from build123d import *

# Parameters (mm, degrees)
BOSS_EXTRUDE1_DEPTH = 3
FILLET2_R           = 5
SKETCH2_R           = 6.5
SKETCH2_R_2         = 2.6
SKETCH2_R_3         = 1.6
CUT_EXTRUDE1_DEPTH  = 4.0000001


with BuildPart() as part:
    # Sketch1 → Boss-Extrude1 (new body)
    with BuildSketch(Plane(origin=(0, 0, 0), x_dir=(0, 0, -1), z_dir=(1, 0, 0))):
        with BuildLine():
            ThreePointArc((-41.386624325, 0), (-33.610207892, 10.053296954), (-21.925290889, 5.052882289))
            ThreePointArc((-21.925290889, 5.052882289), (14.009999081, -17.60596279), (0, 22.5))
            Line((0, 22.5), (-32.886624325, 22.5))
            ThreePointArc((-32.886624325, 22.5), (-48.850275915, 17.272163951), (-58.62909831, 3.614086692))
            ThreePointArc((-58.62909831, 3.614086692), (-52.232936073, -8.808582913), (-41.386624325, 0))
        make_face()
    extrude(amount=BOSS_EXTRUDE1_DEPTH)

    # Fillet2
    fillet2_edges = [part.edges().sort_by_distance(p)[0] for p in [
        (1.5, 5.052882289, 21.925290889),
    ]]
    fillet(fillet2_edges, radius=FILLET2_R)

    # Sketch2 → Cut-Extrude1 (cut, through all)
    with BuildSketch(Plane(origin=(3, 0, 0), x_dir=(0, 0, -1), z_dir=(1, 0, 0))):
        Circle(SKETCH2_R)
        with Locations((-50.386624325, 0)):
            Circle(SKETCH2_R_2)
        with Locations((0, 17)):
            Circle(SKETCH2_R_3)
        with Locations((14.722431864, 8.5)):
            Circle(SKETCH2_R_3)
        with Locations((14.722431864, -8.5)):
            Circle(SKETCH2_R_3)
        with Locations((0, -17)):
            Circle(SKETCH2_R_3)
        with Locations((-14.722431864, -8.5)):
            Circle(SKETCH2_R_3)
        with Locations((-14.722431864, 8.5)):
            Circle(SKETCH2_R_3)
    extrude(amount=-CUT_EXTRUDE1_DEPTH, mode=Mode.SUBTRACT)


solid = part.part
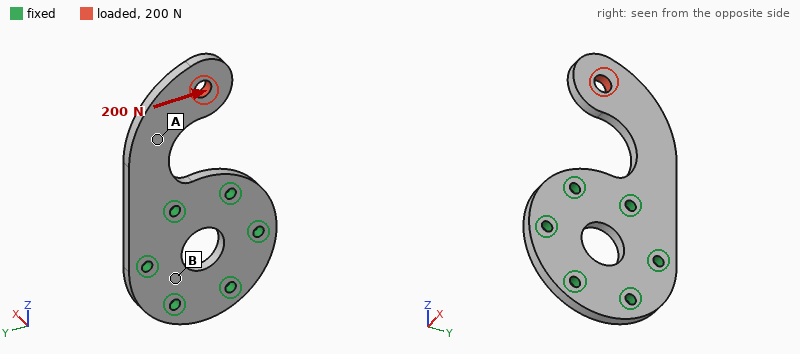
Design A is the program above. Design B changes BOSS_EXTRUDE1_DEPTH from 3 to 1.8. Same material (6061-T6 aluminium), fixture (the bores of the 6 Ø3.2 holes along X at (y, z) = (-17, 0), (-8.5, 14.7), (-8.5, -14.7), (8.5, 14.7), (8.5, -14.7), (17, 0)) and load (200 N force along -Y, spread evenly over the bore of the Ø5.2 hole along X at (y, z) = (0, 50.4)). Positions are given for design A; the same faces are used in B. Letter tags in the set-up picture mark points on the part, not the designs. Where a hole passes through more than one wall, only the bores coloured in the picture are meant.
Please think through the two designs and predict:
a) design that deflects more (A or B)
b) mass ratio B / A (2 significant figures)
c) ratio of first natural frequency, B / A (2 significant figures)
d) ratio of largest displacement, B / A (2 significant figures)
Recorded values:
B
0.60
0.61
1.7
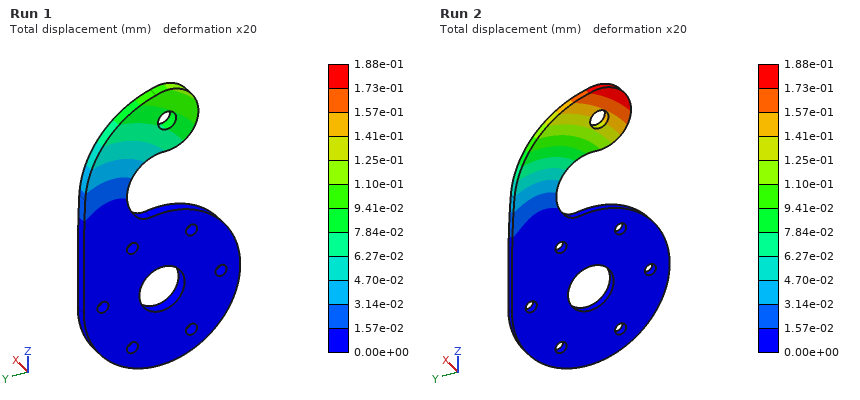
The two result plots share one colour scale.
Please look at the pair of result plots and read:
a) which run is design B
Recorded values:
Run 2
